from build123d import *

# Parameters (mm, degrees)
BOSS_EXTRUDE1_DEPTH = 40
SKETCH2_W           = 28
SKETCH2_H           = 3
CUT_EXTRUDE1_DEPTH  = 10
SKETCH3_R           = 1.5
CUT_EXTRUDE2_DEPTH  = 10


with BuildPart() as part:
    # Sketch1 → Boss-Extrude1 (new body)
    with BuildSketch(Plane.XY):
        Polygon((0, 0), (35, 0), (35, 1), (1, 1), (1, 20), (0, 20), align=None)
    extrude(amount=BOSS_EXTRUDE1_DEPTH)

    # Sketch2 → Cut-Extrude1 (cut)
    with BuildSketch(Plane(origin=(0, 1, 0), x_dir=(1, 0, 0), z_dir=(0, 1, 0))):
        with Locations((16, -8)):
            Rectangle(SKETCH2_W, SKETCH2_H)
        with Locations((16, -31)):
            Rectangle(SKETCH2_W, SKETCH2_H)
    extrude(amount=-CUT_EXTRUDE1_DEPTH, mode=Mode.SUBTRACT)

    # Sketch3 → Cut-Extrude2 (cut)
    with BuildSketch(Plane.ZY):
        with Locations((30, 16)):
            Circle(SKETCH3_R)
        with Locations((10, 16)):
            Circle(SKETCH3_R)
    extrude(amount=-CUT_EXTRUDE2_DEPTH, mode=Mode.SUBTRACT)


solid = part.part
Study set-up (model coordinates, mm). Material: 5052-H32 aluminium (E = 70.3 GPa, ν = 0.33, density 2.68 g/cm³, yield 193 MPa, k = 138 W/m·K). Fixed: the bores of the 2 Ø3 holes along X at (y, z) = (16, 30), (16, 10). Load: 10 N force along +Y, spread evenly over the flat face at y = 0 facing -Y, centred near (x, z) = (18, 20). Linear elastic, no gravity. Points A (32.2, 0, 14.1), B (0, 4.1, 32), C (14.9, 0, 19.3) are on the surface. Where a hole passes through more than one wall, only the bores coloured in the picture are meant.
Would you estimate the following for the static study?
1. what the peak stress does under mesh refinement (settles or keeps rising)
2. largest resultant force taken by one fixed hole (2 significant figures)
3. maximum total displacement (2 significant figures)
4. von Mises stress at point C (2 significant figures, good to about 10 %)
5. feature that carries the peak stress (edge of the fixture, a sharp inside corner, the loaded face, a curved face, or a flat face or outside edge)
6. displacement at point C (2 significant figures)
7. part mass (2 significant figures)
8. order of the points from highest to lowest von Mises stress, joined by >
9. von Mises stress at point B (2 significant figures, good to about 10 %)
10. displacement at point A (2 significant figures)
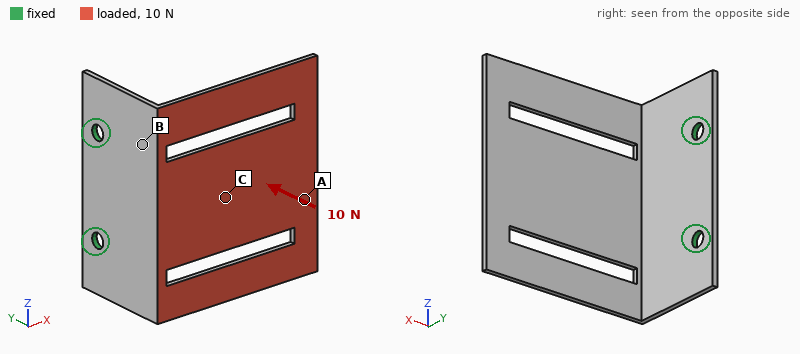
keeps rising
5.1 N
0.61 mm
10 MPa
edge of the fixture
0.23 mm
5.3 g
B > C > A
21 MPa
0.56 mm
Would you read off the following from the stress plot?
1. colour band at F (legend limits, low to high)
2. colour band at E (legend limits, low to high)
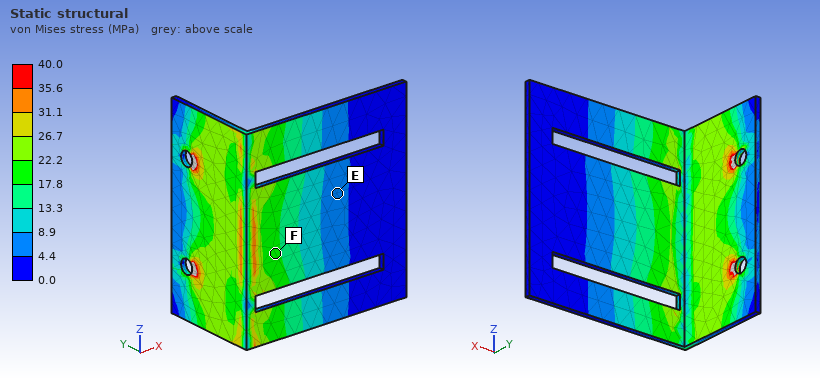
17.8 to 22.2 MPa
4.4 to 8.9 MPa
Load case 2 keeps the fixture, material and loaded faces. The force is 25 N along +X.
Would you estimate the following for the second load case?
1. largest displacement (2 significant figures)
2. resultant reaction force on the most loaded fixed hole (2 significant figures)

0.50 mm
13 N
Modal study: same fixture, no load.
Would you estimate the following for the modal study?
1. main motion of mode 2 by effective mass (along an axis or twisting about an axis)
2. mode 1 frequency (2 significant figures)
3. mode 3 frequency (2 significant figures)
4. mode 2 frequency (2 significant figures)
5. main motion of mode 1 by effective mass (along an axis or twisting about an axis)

along Z
420 Hz
1400 Hz
880 Hz
along Y
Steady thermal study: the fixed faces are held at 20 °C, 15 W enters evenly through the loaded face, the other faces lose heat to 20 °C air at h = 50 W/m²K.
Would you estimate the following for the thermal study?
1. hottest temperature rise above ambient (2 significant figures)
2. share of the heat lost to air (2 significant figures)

70 K
36 %
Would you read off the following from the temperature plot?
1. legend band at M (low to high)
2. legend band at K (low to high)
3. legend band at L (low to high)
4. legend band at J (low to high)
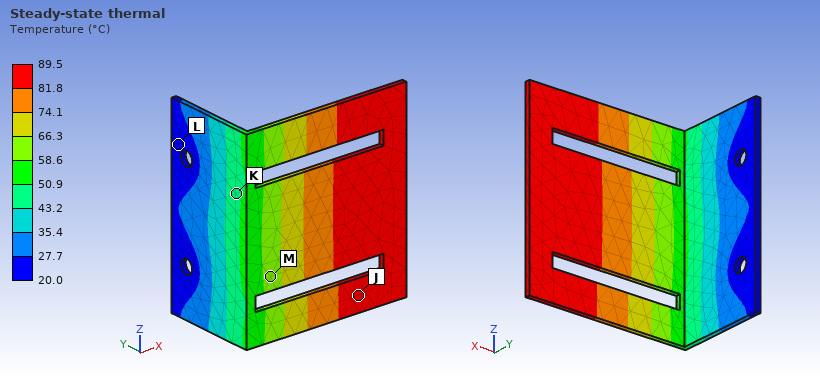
58.6 to 66.3 °C
43.2 to 50.9 °C
20.0 to 27.7 °C
81.8 to 89.5 °C
